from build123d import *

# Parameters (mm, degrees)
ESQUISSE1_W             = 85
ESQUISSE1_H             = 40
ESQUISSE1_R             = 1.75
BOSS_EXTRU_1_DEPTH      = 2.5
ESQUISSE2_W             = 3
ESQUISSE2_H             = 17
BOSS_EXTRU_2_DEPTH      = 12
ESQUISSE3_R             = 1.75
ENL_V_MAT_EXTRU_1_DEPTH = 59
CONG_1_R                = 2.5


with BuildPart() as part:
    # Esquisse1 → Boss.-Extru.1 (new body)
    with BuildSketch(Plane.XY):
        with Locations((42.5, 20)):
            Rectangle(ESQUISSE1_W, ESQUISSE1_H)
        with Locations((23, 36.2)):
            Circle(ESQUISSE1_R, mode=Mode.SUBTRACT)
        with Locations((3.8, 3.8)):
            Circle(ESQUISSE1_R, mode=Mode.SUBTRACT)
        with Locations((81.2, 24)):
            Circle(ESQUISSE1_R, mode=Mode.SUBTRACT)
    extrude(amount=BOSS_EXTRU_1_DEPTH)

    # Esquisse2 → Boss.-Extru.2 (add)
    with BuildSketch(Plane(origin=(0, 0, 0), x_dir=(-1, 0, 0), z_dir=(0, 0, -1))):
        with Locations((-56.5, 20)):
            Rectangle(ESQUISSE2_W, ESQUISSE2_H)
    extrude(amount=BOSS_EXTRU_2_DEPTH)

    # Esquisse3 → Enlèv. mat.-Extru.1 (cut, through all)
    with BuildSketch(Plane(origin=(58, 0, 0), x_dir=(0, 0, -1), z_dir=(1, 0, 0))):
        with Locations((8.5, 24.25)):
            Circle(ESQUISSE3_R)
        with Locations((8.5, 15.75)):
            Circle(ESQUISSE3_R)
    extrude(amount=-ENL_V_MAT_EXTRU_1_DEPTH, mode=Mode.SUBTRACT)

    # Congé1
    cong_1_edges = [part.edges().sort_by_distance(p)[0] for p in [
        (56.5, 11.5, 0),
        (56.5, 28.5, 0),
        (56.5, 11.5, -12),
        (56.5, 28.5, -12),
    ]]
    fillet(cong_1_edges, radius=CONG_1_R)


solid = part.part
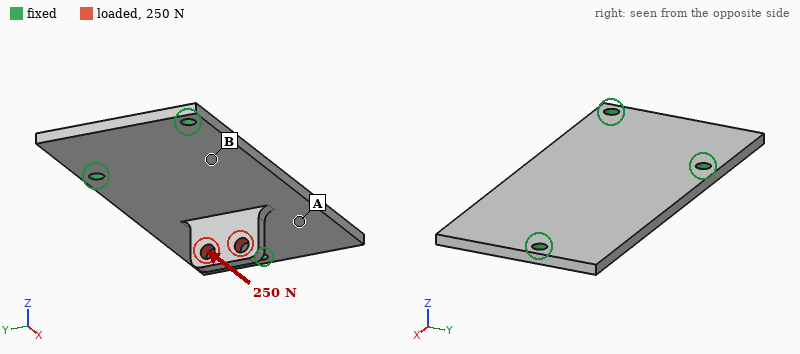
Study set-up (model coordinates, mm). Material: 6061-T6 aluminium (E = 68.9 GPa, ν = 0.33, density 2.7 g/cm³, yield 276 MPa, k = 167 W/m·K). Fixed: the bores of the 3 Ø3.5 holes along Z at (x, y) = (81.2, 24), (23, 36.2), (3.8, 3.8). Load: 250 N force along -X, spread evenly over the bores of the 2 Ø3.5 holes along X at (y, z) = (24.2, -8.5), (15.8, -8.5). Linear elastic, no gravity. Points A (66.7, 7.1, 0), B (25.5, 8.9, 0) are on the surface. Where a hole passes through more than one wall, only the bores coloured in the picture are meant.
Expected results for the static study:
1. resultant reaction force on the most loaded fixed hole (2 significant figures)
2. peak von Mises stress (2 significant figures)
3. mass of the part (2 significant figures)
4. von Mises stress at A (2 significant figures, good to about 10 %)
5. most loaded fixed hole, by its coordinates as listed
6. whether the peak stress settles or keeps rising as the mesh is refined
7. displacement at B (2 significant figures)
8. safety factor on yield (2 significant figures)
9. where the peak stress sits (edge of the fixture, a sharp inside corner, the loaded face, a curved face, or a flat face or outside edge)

130 N
100 MPa
24 g
13 MPa
(81.2, 24)
settles
22 µm
2.7
a curved face
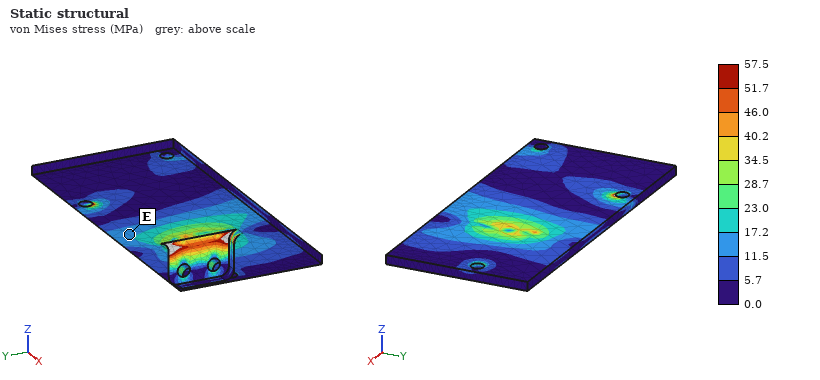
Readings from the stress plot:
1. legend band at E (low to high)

11.5 to 17.2 MPa
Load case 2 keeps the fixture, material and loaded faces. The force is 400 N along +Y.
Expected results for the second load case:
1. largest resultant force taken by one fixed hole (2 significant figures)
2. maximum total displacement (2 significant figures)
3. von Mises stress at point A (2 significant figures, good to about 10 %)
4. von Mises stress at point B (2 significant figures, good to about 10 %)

200 N
0.23 mm
15 MPa
28 MPa
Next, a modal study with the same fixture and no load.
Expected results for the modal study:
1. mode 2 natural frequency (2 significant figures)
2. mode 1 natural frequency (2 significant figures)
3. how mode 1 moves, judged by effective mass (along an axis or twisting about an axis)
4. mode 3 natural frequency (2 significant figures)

3500 Hz
2000 Hz
along Z
4700 Hz
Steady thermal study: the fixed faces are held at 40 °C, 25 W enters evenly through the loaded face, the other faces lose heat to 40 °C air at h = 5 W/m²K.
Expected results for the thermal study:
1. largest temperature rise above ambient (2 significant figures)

65 K
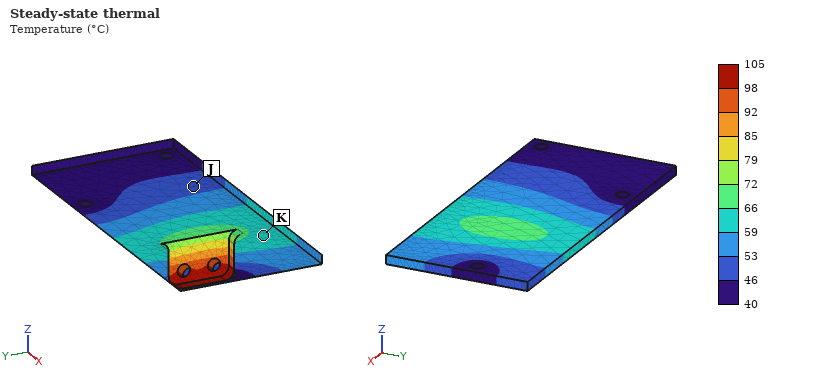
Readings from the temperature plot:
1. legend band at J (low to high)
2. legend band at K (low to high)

46 to 53 °C
59 to 66 °C
